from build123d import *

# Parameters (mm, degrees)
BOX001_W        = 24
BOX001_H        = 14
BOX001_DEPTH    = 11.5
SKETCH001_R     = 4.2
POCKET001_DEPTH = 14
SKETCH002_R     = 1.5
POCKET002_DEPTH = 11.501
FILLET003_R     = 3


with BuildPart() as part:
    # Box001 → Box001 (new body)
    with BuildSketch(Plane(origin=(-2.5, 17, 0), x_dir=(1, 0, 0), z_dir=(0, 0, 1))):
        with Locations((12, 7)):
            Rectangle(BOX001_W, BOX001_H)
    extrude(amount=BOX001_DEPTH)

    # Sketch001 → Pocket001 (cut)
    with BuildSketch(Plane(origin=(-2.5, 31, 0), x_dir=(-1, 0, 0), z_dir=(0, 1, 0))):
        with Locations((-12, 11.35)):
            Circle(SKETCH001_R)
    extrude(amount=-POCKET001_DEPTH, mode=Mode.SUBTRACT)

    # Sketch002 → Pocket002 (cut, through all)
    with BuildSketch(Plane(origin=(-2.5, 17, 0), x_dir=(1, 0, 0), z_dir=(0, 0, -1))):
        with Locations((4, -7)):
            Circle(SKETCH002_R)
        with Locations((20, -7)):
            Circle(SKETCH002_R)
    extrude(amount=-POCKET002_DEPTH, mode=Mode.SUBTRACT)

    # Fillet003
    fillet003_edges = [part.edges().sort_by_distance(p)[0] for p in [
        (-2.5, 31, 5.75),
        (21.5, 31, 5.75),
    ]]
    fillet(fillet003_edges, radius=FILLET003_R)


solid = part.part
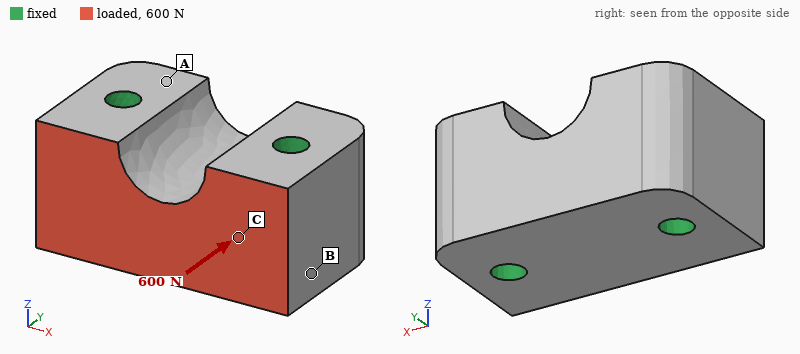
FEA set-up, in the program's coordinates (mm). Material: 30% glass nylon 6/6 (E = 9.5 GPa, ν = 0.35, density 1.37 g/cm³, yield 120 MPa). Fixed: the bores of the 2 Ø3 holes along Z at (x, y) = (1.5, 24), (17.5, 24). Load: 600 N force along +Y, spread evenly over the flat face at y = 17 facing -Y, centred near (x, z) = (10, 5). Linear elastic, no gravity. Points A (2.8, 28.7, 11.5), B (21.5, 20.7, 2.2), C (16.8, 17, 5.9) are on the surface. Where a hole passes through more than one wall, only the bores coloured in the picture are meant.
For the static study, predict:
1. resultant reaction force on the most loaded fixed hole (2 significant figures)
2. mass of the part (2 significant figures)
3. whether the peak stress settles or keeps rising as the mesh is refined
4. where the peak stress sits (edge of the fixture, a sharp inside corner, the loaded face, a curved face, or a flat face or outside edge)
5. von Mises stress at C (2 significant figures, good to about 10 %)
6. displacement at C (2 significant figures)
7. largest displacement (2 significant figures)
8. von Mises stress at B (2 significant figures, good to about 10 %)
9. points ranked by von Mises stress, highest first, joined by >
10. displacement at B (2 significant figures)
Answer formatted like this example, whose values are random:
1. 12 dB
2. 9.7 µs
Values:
1. 300 N
2. 4.5 g
3. keeps rising
4. edge of the fixture
5. 2.9 MPa
6. 1.8 µm
7. 3.6 µm
8. 1.5 MPa
9. C > B > A
10. 1.2 µm
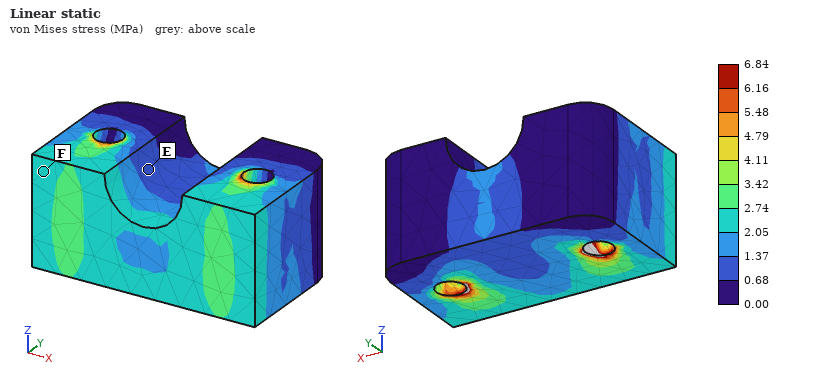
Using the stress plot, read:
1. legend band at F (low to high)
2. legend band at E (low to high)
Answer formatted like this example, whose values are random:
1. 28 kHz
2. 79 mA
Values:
1. 2.05 to 2.74 MPa
2. 0.68 to 1.37 MPa
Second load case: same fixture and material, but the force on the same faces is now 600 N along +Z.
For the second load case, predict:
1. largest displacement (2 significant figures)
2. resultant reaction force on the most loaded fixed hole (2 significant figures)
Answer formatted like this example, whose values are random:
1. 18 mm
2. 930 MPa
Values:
1. 13 µm
2. 300 N
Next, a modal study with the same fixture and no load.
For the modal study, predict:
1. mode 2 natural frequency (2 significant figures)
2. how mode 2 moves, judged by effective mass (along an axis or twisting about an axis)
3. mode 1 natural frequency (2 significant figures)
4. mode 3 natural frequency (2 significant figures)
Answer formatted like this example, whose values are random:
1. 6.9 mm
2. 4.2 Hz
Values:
1. 40 kHz
2. along Z
3. 37 kHz
4. 43 kHz
